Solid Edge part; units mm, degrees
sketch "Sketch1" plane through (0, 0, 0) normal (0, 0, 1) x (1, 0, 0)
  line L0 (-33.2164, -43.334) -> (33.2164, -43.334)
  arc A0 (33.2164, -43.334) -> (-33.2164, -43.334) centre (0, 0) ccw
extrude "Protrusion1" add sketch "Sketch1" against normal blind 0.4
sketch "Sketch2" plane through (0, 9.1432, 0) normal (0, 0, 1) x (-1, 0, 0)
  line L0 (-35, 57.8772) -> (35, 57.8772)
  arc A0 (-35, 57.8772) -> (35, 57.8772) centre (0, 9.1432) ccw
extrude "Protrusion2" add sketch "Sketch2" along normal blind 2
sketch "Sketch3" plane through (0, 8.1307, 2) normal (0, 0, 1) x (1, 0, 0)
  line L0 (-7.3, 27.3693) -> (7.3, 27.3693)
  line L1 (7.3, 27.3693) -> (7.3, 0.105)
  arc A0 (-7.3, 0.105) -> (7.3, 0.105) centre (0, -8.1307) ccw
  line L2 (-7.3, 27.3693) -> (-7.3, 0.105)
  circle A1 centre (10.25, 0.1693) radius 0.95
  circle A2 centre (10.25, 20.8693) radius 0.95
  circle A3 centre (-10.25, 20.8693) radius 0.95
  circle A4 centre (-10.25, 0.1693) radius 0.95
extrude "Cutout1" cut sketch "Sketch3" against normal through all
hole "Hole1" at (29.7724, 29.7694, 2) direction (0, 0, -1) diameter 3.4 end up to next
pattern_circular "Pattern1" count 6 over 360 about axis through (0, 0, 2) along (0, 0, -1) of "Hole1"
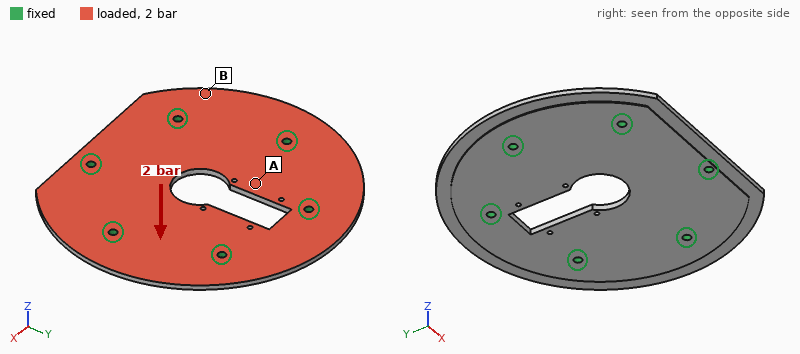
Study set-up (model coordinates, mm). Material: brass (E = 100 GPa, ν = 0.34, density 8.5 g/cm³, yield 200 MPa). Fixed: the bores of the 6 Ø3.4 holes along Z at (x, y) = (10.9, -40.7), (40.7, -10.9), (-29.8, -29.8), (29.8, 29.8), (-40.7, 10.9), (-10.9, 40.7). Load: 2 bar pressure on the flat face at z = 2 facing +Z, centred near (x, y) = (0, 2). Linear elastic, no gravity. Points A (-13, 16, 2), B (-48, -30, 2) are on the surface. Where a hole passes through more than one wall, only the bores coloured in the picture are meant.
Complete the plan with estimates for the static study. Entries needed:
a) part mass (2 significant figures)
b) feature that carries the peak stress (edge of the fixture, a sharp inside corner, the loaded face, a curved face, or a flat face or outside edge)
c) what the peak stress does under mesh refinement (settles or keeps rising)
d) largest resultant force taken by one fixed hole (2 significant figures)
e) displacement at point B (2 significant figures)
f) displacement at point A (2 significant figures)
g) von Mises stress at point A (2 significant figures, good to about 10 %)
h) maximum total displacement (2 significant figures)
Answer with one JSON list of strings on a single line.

["200 g", "edge of the fixture", "keeps rising", "360 N", "31 µm", "47 µm", "19 MPa", "76 µm"]
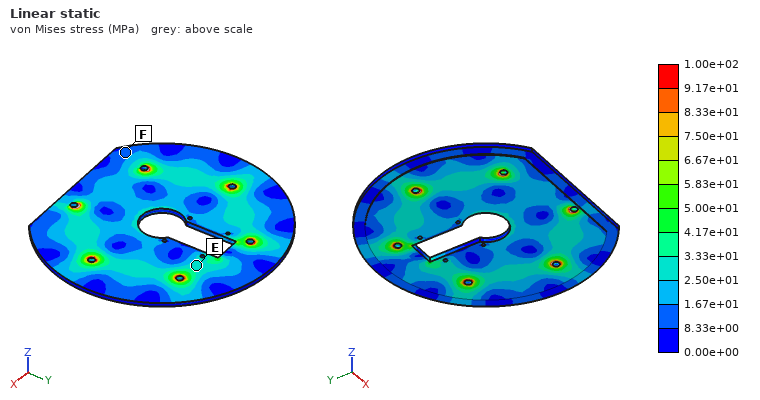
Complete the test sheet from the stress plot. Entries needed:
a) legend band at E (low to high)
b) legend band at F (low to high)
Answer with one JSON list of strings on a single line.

["2.50e+01 to 3.33e+01 MPa", "8.33e+00 to 1.67e+01 MPa"]
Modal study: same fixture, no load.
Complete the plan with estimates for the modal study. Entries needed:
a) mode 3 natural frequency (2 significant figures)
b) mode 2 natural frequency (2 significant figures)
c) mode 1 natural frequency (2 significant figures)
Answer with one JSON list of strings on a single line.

["2400 Hz", "2300 Hz", "2000 Hz"]
